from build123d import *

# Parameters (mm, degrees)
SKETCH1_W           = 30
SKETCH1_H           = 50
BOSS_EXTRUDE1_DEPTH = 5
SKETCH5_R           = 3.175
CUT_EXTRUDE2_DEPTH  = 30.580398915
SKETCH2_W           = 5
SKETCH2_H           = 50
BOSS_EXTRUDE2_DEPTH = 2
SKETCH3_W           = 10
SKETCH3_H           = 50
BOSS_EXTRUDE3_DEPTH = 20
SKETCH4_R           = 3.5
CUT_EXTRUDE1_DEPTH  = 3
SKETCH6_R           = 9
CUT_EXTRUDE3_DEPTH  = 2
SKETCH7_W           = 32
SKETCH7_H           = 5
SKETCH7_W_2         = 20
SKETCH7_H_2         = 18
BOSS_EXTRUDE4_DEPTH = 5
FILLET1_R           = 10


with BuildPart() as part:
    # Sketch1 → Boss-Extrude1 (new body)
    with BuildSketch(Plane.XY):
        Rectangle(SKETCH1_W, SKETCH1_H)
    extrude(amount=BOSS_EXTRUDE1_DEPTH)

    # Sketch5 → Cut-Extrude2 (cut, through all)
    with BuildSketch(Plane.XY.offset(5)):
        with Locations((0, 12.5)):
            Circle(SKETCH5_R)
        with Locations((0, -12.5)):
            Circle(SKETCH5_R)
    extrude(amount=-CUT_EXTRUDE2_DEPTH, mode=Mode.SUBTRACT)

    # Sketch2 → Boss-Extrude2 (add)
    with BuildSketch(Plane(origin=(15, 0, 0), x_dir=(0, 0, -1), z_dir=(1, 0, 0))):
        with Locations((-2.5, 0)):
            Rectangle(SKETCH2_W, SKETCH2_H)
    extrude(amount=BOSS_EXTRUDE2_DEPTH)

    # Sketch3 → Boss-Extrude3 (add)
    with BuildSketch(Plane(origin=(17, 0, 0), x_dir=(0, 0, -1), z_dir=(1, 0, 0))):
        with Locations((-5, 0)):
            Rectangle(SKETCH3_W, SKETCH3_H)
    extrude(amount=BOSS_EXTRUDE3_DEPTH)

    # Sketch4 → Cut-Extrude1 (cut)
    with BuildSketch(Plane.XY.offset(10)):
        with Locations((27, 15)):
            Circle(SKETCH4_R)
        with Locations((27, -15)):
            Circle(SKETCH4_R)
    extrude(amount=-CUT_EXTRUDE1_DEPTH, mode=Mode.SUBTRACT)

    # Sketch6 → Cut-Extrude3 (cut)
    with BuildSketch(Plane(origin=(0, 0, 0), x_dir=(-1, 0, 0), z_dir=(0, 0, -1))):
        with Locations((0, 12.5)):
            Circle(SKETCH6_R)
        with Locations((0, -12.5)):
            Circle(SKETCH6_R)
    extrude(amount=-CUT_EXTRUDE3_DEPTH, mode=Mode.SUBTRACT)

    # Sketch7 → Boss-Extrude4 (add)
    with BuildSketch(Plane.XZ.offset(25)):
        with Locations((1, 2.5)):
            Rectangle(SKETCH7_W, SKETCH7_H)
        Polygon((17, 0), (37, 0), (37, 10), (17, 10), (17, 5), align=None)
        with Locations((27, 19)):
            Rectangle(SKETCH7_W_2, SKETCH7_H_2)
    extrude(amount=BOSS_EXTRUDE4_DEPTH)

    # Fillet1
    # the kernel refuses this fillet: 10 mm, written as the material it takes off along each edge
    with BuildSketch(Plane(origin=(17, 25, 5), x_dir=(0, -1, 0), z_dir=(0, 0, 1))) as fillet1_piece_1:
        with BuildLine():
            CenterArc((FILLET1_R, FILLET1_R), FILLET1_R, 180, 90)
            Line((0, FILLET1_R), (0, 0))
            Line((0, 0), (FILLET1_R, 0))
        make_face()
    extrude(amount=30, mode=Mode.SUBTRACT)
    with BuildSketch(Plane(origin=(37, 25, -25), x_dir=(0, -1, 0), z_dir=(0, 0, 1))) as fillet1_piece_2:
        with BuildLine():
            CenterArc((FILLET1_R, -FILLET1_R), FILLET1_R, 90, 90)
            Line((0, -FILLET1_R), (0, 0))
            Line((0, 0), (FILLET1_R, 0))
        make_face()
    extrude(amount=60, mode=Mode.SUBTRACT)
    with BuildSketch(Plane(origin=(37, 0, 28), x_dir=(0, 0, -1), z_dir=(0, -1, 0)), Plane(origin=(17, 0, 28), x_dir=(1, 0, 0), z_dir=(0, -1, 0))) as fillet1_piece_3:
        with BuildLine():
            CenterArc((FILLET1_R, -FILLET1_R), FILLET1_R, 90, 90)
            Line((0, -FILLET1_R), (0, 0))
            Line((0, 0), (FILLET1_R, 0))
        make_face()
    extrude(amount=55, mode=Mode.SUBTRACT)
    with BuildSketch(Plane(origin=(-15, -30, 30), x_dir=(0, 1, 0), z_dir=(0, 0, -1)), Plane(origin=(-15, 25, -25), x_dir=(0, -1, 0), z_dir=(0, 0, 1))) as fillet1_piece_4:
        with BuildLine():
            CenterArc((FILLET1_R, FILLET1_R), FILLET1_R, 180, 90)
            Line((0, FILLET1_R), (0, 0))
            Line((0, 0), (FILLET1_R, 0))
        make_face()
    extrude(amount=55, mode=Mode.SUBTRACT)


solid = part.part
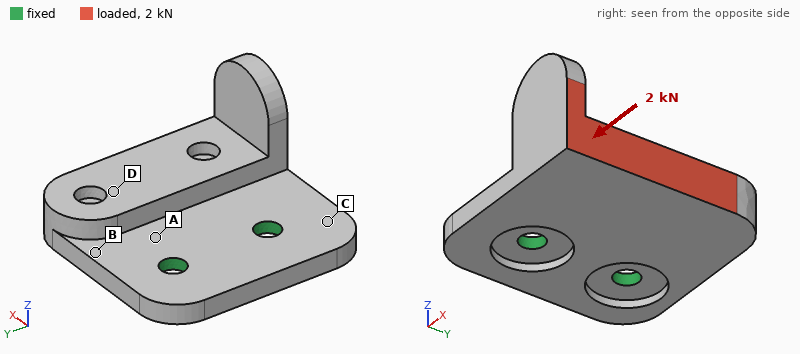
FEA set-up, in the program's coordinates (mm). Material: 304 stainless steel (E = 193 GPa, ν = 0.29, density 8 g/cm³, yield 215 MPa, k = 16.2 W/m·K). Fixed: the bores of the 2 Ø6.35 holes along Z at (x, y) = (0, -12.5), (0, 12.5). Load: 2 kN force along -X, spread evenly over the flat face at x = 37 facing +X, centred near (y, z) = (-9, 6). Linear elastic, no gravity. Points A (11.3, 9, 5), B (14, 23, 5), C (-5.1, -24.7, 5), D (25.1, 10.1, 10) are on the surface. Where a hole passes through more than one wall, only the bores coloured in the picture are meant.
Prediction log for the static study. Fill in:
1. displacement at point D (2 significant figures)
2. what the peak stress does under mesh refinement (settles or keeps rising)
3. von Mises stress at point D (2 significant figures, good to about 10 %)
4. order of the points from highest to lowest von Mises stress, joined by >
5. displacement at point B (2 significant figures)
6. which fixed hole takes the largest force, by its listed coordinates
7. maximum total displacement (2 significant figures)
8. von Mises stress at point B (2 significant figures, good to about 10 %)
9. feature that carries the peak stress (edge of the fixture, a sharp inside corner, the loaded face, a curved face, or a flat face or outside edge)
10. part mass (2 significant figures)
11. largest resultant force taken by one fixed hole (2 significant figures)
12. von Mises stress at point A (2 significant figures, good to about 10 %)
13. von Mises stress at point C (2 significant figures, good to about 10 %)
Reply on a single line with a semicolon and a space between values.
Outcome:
25 µm; keeps rising; 6.1 MPa; A > B > C > D; 8.6 µm; (0, -12.5); 53 µm; 21 MPa; edge of the fixture; 160 g; 1.6 kN; 28 MPa; 12 MPa
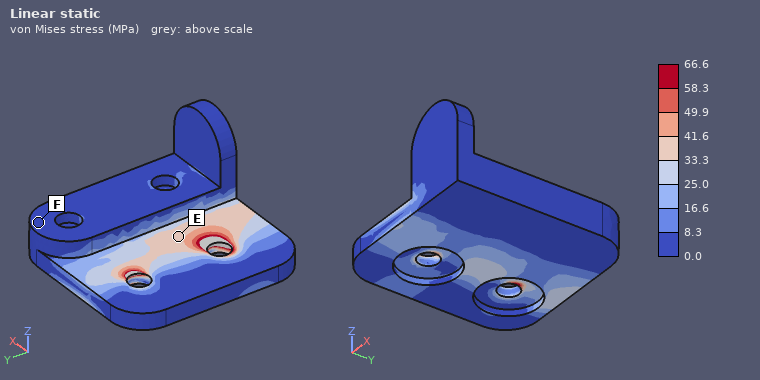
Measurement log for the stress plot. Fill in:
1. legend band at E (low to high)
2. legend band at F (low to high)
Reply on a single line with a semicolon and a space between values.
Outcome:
33.3 to 41.6 MPa; 0.0 to 8.3 MPa
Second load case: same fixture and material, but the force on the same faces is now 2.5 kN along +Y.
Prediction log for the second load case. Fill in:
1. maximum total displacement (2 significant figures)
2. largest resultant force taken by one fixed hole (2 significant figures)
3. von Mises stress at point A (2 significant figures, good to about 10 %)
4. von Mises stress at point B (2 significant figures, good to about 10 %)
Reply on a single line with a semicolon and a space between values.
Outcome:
32 µm; 3.4 kN; 62 MPa; 38 MPa
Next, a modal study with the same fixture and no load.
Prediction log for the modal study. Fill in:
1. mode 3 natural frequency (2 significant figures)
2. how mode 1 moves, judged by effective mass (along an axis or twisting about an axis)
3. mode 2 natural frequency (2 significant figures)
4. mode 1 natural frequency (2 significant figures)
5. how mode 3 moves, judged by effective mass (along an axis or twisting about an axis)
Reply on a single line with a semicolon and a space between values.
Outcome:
7200 Hz; along Z; 3400 Hz; 1400 Hz; along Y
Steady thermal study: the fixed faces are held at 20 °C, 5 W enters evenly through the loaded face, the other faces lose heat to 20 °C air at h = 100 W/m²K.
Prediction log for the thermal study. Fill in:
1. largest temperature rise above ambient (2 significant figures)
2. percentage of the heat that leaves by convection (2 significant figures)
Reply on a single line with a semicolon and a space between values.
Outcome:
16 K; 82 %
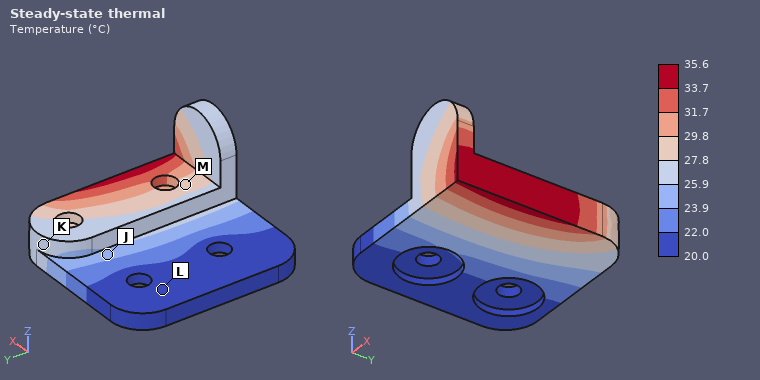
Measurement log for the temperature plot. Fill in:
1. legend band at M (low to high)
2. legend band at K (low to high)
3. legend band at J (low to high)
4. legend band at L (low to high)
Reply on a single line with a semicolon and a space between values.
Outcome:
27.8 to 29.8 °C; 25.9 to 27.8 °C; 23.9 to 25.9 °C; 20.0 to 22.0 °C
